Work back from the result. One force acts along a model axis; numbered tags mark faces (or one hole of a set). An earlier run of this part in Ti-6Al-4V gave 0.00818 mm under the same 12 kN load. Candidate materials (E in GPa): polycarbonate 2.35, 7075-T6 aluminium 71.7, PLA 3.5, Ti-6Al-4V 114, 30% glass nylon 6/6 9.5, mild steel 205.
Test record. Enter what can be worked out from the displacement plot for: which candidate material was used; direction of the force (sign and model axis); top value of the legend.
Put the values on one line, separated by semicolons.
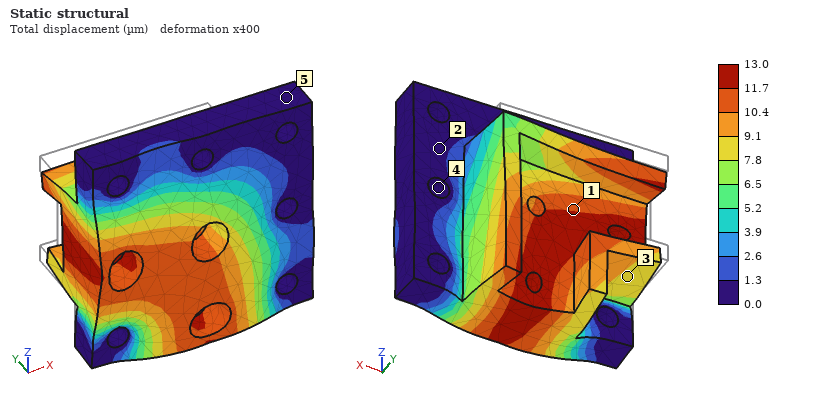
7075-T6 aluminium; -Y; 13.0 µm
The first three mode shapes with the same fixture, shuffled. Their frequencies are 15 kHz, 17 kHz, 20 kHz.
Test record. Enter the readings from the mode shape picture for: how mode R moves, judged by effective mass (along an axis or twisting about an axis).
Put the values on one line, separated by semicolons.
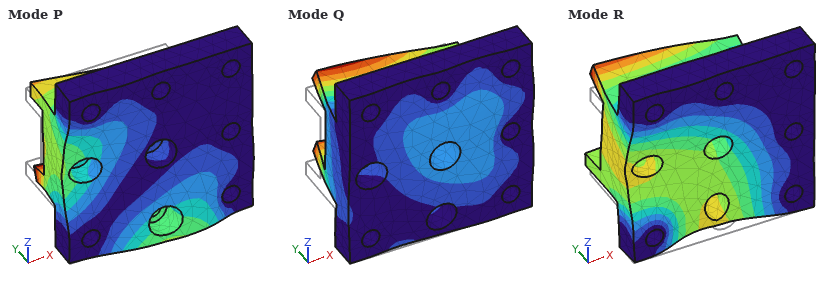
along Y
